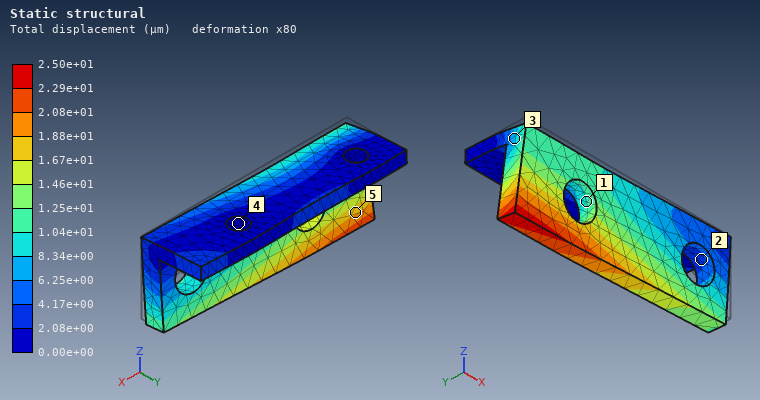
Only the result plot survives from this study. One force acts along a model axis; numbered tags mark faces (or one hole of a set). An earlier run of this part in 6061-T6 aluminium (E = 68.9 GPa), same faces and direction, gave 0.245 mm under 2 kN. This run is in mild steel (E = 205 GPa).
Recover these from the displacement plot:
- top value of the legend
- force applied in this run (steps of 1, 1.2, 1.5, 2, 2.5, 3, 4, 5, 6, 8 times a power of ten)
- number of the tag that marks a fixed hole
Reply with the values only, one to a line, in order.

2.50e+01 µm
600 N
4
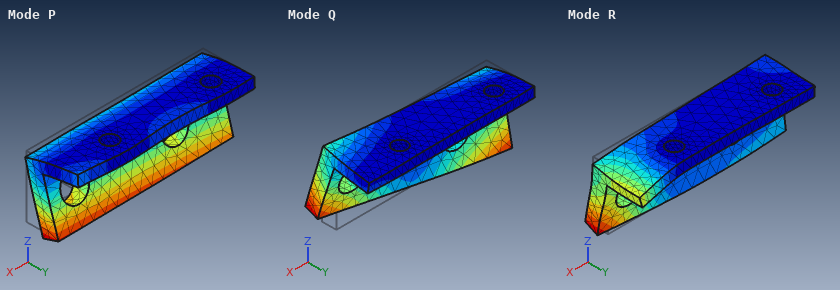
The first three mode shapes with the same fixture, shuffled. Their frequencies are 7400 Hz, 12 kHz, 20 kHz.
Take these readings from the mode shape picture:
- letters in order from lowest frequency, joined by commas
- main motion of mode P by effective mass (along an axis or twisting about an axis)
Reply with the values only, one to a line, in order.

P, Q, R
along Y
